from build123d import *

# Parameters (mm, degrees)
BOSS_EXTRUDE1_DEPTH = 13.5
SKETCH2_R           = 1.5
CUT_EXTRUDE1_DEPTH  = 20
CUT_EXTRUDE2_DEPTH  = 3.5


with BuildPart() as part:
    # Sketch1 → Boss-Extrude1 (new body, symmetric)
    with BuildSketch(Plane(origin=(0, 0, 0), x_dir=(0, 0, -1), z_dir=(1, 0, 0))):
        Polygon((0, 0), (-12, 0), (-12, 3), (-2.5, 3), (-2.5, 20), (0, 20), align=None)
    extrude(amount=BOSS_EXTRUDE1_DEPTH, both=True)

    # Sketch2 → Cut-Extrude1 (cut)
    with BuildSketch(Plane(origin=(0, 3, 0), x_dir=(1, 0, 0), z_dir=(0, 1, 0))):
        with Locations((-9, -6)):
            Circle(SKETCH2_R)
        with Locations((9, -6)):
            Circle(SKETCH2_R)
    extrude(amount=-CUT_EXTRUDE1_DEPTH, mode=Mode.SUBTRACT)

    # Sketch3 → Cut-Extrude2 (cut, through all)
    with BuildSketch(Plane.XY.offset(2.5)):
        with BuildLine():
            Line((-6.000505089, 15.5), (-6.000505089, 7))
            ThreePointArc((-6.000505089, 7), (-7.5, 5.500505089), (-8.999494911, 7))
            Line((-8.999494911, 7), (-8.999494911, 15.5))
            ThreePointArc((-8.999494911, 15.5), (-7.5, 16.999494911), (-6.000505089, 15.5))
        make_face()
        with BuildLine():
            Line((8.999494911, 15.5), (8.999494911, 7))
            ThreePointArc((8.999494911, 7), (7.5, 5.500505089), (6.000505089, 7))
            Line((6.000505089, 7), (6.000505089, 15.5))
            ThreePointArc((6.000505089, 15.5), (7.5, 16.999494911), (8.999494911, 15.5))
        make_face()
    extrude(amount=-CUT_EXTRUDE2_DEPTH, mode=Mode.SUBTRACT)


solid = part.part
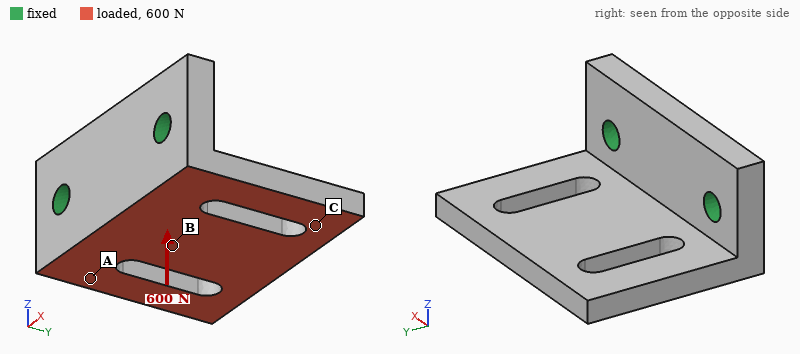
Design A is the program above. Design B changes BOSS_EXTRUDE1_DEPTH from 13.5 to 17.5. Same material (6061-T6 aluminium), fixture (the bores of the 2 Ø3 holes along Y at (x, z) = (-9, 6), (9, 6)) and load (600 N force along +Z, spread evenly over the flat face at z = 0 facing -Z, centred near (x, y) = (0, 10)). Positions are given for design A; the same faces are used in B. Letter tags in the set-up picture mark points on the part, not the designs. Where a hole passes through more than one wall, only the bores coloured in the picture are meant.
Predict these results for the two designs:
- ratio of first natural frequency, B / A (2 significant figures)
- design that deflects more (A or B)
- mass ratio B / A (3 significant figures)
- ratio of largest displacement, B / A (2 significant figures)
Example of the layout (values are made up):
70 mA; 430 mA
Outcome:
0.98; A; 1.33; 0.78
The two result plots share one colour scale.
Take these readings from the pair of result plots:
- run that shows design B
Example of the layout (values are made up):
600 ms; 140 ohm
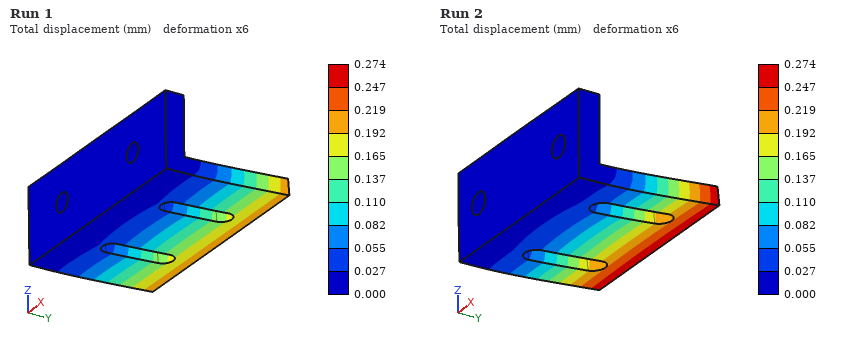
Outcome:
Run 1
